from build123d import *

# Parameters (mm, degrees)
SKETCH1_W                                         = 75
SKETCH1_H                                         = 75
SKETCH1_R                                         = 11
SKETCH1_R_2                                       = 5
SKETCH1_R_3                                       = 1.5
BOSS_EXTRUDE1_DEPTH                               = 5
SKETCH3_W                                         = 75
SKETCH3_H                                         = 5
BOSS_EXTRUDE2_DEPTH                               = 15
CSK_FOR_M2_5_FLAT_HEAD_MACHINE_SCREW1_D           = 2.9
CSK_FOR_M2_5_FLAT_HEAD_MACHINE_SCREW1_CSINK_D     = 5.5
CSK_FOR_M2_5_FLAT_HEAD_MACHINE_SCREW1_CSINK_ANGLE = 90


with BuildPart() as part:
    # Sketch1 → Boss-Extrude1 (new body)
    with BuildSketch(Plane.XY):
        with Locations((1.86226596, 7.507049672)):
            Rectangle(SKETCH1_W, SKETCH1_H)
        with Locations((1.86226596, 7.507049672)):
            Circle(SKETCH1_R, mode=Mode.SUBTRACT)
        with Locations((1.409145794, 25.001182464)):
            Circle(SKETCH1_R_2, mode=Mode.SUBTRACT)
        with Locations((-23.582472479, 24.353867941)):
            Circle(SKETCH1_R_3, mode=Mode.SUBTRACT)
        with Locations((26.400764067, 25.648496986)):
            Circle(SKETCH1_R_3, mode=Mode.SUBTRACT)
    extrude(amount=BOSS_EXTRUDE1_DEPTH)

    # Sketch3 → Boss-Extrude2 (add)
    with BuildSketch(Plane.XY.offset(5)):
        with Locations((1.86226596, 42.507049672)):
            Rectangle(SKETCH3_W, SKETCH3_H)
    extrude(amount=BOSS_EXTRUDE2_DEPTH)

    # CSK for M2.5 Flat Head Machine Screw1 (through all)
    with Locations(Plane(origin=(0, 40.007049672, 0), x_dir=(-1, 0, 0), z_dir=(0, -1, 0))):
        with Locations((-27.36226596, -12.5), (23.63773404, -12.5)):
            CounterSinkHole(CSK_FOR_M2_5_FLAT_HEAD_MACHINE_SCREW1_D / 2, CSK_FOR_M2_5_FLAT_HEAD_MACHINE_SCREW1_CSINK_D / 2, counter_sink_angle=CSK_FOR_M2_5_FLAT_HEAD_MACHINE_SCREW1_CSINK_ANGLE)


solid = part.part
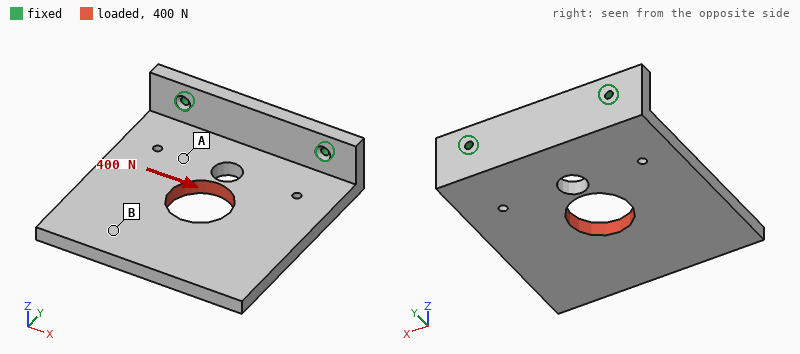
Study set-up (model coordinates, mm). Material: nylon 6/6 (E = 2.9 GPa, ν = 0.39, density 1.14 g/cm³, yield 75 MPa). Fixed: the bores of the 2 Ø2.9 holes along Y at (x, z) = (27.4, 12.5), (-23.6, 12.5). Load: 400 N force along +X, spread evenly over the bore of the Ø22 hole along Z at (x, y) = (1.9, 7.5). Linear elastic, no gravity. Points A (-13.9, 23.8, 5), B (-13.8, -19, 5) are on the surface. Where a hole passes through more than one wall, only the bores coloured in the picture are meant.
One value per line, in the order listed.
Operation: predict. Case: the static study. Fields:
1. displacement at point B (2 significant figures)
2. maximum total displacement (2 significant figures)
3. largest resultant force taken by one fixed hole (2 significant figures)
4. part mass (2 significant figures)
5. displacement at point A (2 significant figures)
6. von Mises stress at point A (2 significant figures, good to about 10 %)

0.63 mm
0.88 mm
340 N
36 g
0.25 mm
5.4 MPa
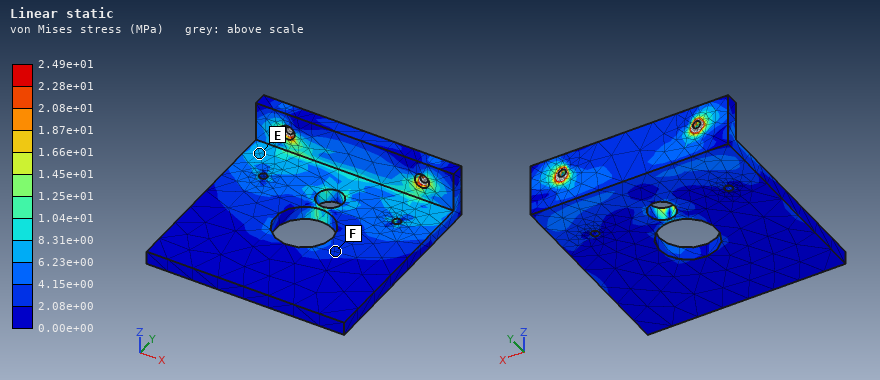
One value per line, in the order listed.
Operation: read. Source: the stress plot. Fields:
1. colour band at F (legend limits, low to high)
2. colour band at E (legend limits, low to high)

2.08e+00 to 4.15e+00 MPa
6.23e+00 to 8.31e+00 MPa
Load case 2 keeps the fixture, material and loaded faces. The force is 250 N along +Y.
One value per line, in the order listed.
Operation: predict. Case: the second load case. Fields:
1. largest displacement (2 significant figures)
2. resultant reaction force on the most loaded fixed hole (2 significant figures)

1.2 mm
130 N
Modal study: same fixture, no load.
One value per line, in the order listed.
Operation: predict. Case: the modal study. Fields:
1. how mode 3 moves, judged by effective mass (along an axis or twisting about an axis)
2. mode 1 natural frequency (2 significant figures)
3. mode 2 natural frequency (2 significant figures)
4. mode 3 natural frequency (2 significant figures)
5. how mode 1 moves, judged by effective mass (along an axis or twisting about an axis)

along X
170 Hz
470 Hz
850 Hz
along Z
